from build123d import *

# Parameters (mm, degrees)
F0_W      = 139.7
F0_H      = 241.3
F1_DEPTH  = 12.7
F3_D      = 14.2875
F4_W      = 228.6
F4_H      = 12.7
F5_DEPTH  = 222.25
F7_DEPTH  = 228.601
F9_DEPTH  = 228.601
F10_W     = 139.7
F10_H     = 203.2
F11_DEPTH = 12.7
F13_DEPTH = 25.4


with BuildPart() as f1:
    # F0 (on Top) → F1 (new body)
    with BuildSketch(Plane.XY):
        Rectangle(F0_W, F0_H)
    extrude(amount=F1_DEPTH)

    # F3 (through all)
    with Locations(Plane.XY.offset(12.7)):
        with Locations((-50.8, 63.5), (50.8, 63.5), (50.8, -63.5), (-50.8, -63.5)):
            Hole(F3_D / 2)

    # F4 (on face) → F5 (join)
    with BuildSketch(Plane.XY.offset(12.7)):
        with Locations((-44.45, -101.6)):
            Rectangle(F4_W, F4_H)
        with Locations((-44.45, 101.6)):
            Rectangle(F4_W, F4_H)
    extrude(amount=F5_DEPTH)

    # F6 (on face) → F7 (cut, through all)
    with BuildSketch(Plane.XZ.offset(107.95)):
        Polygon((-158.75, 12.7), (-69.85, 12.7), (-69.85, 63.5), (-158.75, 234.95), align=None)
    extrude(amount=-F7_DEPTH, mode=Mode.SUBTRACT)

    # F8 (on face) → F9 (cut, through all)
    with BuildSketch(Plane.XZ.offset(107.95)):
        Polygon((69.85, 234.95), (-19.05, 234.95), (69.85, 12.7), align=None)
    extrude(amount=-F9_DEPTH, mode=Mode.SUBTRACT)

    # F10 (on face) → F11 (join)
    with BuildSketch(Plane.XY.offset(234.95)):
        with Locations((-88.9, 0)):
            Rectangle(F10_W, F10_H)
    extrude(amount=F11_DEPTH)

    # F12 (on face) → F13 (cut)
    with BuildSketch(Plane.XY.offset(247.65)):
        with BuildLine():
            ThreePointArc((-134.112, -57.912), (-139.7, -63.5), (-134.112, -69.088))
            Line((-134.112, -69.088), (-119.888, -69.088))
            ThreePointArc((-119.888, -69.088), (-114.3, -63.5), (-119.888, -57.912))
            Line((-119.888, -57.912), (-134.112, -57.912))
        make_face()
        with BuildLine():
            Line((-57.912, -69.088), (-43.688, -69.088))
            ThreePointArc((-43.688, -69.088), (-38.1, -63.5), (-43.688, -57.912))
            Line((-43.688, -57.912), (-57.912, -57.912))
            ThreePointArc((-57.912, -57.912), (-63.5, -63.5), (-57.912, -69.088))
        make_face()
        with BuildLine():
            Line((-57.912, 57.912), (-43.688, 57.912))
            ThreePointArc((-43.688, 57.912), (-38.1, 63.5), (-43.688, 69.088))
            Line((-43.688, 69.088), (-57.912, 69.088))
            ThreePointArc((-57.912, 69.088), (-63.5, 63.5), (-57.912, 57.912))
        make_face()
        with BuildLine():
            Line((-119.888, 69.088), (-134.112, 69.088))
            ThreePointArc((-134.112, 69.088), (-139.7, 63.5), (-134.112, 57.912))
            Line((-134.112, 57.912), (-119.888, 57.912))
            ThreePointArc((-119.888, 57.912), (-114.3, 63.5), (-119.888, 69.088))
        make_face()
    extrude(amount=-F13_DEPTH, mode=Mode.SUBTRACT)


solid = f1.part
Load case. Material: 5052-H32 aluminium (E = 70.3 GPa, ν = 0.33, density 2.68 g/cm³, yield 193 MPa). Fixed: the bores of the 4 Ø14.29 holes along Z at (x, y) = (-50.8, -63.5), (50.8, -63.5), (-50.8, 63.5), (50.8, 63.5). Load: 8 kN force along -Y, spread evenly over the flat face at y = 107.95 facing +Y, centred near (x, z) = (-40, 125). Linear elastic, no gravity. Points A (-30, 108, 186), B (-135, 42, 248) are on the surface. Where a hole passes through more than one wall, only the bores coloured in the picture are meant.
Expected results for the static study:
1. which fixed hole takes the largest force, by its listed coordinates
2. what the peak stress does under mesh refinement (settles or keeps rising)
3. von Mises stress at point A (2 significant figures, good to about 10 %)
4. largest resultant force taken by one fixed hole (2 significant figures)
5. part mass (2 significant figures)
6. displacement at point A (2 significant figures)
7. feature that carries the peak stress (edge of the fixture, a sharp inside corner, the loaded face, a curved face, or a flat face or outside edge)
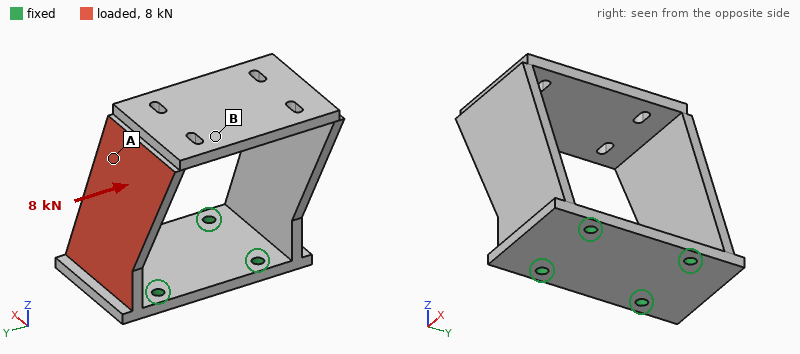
(-50.8, 63.5)
keeps rising
47 MPa
4.4 kN
4.0 kg
2.7 mm
edge of the fixture
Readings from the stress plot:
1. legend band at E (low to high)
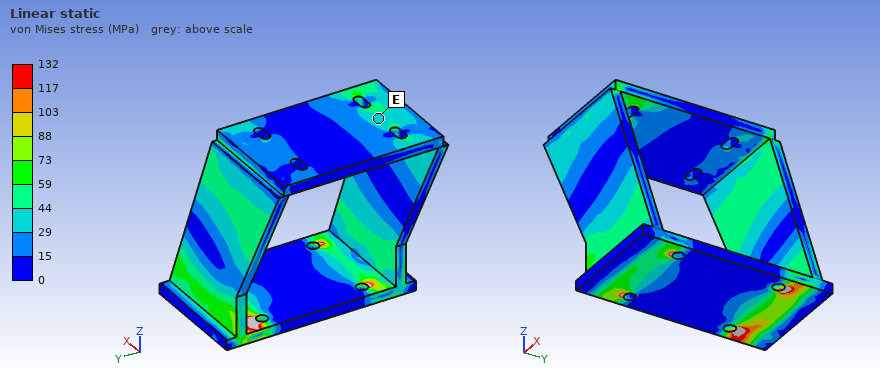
29 to 44 MPa
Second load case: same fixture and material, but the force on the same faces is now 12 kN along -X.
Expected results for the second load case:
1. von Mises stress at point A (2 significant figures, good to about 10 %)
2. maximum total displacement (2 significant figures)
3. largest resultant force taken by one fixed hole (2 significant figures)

20 MPa
1.1 mm
15 kN
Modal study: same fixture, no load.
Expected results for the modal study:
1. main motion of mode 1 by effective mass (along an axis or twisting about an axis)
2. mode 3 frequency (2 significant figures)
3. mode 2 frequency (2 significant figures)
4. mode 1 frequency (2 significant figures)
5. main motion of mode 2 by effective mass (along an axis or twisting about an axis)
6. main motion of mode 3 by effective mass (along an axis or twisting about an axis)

along Y
540 Hz
390 Hz
140 Hz
along X
twisting about Z
